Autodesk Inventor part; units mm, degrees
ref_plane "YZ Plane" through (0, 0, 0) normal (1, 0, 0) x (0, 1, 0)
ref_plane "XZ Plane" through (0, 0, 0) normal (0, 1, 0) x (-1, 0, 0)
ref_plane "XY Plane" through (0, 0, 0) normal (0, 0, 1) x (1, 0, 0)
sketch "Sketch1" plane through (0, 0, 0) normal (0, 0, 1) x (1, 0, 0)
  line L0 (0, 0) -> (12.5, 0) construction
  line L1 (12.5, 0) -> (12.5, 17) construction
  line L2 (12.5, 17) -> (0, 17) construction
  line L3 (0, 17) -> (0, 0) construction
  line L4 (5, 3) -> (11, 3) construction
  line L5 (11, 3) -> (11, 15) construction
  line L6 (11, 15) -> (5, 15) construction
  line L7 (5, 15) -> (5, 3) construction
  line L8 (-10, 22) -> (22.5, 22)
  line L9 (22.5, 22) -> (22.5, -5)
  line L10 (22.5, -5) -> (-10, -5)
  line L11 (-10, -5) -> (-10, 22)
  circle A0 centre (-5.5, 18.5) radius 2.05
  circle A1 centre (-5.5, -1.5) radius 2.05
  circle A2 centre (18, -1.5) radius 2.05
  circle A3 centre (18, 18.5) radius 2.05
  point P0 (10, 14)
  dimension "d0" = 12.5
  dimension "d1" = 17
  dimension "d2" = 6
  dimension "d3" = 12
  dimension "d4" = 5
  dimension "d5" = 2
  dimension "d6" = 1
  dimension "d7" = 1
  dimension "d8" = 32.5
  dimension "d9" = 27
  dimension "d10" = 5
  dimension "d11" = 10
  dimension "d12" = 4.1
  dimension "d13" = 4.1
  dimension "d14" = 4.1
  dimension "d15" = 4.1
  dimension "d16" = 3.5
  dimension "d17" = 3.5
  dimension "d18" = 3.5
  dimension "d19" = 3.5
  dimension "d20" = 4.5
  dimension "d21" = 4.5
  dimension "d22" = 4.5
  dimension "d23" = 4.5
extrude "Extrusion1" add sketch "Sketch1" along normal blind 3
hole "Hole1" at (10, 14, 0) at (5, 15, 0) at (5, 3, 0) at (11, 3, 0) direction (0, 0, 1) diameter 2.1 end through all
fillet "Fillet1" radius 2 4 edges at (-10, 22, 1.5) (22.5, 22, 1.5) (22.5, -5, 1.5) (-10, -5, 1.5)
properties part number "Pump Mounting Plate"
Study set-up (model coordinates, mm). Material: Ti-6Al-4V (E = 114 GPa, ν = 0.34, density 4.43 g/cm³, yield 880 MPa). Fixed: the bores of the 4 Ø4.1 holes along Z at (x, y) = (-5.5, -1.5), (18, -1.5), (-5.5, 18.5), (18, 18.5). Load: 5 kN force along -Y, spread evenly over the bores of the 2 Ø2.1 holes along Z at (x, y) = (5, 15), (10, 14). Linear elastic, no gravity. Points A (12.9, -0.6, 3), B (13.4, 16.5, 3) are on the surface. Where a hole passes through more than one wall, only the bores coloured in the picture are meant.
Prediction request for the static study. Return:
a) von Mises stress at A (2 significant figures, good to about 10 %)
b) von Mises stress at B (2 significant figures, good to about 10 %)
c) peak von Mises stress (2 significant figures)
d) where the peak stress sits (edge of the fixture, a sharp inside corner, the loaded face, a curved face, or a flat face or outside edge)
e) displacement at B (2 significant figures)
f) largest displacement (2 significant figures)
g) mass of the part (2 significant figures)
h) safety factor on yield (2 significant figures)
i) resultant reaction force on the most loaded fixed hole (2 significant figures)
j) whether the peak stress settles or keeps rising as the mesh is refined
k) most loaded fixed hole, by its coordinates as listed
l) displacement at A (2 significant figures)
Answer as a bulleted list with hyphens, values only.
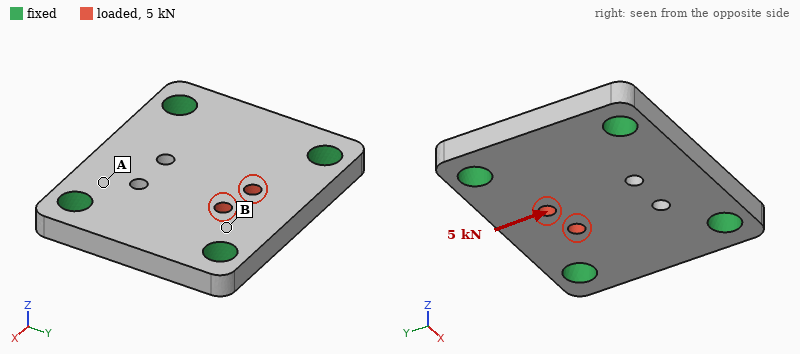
- 34 MPa
- 92 MPa
- 250 MPa
- the loaded face
- 5.1 µm
- 13 µm
- 11 g
- 3.5
- 1.7 kN
- settles
- (18, 18.5)
- 2.4 µm
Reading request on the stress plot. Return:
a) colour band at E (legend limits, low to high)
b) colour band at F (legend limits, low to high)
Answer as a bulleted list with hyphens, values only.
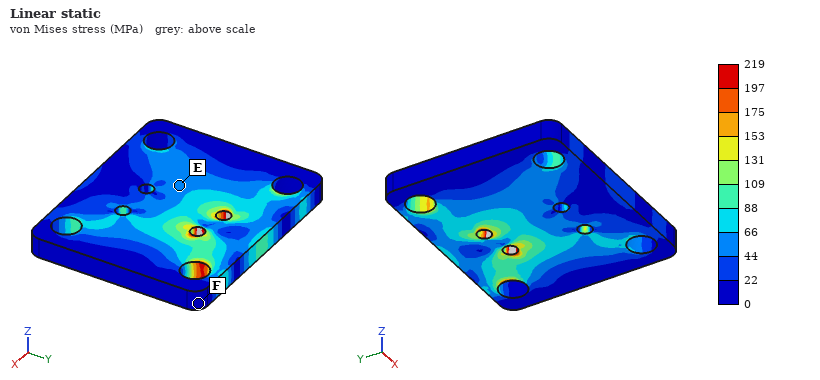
- 44 to 66 MPa
- 0 to 22 MPa
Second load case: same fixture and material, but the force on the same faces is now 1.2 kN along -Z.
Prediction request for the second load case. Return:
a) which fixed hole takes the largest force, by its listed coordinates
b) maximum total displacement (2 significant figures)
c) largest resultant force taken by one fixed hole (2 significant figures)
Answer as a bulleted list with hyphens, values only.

- (18, 18.5)
- 23 µm
- 580 N
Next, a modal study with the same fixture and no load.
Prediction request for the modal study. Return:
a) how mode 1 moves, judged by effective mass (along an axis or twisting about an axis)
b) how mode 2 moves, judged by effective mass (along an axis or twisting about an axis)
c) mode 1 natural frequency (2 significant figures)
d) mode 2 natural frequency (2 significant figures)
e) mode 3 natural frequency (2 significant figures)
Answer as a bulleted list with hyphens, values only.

- along Z
- twisting about X
- 26 kHz
- 36 kHz
- 41 kHz
